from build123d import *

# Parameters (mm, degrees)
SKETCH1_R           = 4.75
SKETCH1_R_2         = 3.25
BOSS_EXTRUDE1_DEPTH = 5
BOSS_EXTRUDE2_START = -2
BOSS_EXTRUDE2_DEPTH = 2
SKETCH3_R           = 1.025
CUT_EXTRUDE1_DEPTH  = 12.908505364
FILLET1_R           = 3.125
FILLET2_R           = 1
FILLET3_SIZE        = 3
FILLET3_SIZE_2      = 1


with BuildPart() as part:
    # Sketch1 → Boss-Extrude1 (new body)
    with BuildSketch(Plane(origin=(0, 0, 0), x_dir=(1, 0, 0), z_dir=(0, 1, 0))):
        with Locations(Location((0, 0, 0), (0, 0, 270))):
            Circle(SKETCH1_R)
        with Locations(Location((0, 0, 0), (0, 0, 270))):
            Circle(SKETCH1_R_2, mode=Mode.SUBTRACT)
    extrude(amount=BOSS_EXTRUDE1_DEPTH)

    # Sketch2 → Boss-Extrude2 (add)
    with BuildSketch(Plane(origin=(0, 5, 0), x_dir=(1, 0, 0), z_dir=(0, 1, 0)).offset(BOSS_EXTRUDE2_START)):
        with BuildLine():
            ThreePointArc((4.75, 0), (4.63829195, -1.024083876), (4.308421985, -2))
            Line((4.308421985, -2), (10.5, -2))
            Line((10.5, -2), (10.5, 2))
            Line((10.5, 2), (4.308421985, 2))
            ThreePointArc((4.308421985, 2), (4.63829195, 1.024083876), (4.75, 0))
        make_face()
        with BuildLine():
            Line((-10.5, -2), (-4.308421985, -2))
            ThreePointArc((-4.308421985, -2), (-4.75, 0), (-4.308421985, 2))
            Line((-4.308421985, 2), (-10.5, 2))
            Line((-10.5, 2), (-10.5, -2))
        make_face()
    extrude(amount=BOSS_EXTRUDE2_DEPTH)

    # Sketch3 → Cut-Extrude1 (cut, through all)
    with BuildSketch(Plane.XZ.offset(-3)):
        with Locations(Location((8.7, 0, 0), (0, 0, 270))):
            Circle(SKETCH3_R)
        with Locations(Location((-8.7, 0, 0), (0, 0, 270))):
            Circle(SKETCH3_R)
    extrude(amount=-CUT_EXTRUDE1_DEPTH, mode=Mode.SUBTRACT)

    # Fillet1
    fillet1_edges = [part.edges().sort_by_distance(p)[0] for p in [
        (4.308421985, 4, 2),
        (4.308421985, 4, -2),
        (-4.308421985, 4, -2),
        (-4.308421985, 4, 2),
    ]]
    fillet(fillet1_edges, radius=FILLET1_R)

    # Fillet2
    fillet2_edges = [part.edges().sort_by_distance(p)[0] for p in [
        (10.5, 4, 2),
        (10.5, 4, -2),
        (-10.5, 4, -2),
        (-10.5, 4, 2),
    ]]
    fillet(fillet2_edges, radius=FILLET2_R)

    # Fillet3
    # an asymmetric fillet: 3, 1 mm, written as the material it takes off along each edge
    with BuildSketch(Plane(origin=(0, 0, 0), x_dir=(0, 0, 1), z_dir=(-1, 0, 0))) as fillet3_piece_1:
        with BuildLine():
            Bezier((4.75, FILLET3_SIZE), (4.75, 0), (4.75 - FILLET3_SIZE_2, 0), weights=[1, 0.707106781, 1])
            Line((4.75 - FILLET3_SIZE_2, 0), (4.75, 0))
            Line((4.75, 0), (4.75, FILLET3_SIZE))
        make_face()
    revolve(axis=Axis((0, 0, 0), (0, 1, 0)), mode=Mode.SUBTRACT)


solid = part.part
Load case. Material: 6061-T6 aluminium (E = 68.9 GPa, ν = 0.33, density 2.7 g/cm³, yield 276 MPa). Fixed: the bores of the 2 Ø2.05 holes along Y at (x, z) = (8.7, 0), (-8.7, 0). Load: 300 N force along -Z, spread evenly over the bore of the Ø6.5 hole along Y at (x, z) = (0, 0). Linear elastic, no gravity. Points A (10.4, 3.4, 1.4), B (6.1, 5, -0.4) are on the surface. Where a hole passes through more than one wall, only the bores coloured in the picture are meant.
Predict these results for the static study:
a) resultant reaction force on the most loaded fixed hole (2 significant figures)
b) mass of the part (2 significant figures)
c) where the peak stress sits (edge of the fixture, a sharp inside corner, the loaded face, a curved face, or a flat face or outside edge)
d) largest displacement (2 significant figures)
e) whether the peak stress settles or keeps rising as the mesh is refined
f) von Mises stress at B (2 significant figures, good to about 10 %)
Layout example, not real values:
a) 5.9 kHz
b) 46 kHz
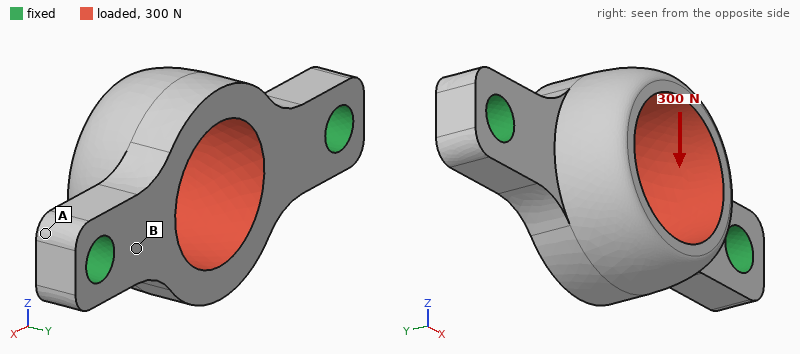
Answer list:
a) 150 N
b) 0.68 g
c) edge of the fixture
d) 30 µm
e) keeps rising
f) 33 MPa
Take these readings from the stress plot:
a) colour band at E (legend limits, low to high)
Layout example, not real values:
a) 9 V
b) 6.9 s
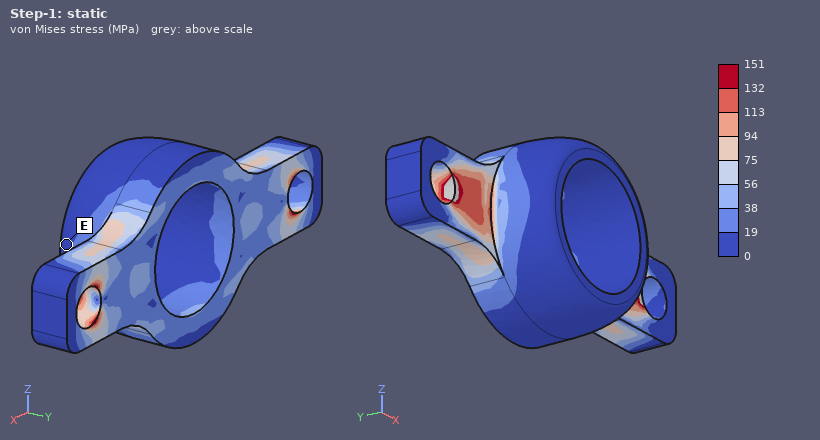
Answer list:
a) 0 to 19 MPa
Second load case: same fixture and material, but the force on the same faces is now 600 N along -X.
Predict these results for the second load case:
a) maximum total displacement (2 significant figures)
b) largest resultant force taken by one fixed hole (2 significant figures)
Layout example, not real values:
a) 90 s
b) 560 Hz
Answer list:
a) 7.3 µm
b) 310 N
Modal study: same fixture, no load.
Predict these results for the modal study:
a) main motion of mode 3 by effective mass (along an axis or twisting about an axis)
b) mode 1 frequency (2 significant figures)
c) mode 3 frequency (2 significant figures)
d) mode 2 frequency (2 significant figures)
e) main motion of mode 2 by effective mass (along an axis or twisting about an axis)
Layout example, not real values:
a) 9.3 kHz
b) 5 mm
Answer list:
a) along Z
b) 22 kHz
c) 54 kHz
d) 31 kHz
e) along Y
